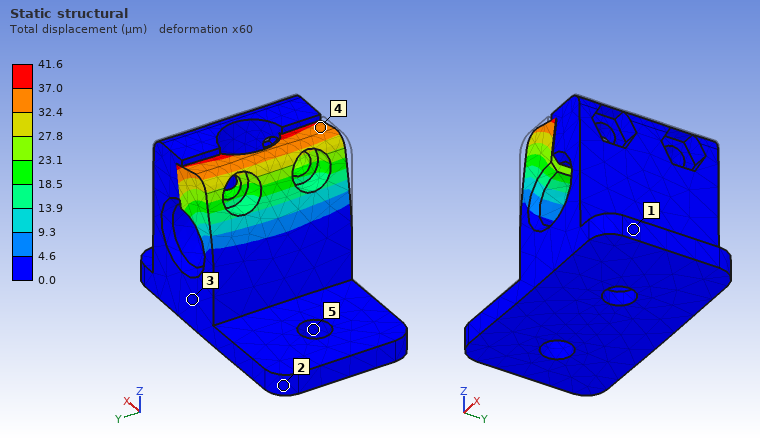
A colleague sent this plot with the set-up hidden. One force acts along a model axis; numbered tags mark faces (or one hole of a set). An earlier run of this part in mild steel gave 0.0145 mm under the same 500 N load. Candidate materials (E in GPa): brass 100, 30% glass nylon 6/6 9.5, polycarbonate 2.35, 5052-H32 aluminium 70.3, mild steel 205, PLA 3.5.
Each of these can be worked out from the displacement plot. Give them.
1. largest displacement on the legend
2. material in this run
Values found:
41.6 µm
5052-H32 aluminium
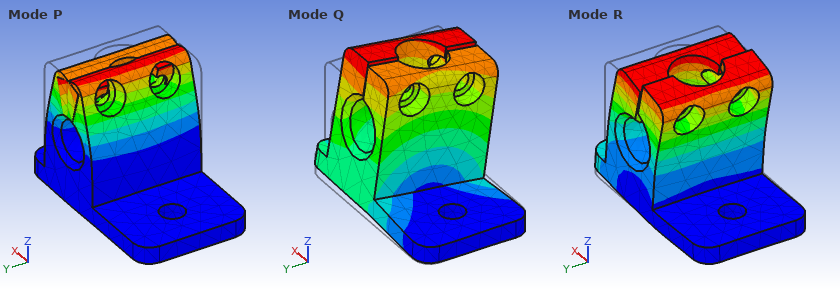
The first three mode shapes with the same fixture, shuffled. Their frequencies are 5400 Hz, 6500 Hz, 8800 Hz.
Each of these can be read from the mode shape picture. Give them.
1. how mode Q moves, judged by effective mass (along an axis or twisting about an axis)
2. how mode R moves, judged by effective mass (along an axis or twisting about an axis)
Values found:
along Y
along X
